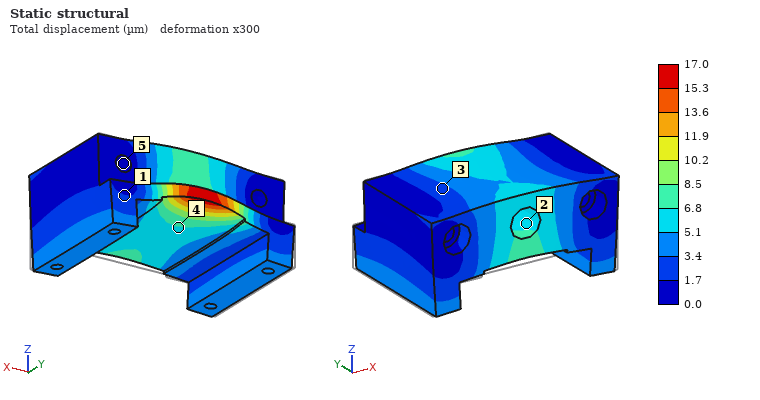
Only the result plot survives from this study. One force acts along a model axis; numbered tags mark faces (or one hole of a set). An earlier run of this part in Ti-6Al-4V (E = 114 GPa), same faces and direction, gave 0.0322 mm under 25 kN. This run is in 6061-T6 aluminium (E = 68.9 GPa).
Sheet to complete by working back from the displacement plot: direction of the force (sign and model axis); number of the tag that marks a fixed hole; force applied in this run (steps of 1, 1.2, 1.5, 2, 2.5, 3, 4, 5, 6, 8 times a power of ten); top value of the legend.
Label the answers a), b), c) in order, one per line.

a) +Z
b) 5
c) 8 kN
d) 17.0 µm
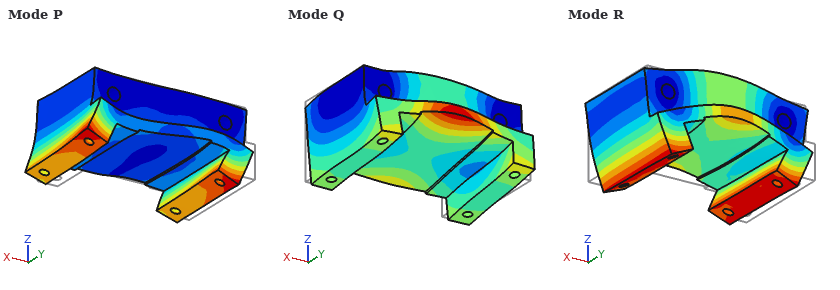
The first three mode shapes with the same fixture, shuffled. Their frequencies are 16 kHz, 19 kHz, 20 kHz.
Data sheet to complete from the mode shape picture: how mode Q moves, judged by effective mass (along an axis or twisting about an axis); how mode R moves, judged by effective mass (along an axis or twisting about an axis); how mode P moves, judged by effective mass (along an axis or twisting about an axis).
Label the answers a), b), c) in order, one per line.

a) along Y
b) along Z
c) along X
